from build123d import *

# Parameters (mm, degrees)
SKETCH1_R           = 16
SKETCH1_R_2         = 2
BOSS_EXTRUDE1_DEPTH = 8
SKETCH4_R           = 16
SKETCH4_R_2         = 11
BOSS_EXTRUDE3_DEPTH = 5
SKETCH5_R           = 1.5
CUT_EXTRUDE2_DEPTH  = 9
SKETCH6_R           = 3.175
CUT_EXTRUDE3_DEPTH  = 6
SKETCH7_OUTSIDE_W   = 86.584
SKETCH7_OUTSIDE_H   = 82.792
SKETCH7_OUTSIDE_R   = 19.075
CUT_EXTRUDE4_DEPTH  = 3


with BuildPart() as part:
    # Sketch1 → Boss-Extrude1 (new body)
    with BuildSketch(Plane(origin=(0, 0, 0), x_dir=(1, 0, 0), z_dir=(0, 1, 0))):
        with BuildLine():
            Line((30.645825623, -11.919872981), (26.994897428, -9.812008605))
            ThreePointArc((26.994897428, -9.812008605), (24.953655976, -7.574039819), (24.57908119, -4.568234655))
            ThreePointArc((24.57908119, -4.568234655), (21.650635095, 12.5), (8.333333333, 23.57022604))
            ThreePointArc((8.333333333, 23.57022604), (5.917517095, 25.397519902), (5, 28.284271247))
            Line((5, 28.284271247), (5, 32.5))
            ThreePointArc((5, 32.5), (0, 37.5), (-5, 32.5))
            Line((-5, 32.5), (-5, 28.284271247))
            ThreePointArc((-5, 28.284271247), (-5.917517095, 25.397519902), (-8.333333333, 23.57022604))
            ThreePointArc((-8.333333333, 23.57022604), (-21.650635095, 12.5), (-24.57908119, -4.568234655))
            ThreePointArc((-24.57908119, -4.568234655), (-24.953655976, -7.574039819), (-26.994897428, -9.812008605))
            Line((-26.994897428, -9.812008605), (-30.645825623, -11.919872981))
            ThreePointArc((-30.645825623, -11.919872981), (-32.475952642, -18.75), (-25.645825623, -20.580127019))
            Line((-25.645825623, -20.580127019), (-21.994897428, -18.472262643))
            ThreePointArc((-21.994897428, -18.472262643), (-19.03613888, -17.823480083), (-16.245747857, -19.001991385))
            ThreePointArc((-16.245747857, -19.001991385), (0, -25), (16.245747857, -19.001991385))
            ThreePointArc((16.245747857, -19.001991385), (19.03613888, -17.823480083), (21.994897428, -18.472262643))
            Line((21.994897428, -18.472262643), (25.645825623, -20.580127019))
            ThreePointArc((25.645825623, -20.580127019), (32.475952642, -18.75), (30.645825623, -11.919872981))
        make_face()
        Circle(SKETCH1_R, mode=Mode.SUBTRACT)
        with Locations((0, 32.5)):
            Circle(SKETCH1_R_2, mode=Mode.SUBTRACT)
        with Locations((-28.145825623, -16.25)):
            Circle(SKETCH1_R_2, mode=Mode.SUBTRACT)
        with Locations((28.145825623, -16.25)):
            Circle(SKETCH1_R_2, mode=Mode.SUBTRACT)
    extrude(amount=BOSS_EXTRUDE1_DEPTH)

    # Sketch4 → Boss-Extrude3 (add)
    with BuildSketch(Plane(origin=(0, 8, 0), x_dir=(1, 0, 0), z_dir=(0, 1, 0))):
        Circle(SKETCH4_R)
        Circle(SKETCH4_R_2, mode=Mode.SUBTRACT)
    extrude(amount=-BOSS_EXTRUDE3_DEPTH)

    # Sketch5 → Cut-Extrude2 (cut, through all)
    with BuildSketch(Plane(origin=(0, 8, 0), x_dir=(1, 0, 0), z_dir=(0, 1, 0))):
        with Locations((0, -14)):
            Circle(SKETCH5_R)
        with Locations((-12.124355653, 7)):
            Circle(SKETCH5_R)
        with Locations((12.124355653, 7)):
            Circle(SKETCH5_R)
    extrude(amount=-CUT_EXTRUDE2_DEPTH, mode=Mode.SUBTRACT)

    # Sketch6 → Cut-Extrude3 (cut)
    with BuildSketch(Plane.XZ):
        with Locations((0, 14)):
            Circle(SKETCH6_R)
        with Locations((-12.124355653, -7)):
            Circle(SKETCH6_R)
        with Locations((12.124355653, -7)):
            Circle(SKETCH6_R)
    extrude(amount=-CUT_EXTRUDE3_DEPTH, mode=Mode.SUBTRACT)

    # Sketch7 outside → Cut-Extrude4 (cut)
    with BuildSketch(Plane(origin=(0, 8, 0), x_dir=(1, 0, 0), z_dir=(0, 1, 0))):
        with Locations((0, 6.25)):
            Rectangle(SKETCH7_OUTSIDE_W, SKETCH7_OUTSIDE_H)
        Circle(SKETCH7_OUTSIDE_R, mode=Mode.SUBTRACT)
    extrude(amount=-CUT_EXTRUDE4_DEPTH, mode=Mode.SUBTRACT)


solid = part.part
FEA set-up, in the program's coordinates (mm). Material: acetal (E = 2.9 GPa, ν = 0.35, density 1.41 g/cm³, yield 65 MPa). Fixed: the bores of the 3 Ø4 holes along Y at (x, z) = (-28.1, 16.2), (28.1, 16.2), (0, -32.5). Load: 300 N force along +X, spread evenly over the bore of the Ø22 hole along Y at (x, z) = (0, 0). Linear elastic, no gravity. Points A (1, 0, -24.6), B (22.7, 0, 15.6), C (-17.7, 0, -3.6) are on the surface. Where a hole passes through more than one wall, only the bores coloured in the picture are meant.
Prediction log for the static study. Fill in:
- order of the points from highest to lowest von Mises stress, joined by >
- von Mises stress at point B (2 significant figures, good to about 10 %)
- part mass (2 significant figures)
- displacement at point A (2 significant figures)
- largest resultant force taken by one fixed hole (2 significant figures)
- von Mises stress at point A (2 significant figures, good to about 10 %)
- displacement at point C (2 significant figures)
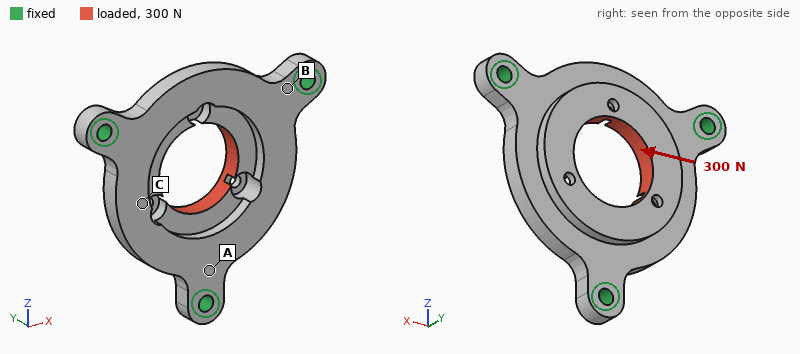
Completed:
B > A > C
3.2 MPa
14 g
21 µm
110 N
1.9 MPa
31 µm
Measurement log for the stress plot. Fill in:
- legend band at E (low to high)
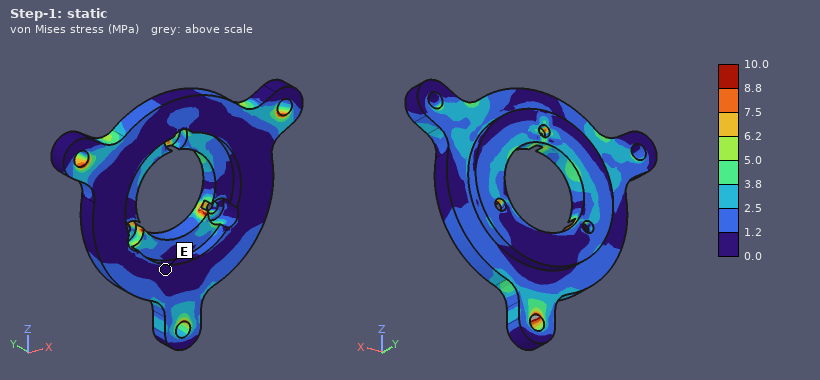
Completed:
0.0 to 1.2 MPa
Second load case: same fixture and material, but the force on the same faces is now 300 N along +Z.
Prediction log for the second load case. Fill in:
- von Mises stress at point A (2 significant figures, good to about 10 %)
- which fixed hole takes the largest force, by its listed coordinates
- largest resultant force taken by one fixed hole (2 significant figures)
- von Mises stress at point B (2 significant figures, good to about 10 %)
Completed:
0.95 MPa
(0, -32.5)
120 N
2.3 MPa
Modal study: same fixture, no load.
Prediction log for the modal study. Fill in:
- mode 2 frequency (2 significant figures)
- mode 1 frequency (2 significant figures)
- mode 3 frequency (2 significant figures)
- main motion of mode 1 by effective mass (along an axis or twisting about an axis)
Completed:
2300 Hz
2100 Hz
2300 Hz
along Y
